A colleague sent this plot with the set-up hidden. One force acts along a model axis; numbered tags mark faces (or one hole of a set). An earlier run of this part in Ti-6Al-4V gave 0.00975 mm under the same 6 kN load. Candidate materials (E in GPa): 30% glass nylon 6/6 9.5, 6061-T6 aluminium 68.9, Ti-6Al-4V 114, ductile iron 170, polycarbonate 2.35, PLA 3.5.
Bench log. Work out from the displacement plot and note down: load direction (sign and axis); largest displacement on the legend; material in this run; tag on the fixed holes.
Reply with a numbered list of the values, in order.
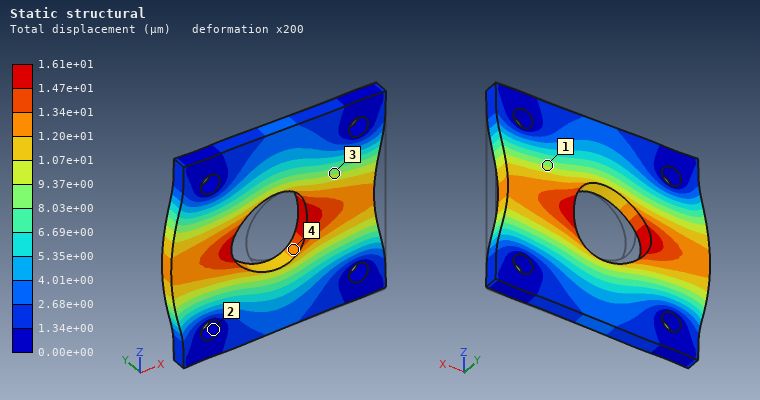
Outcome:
1. -X
2. 1.61e+01 µm
3. 6061-T6 aluminium
4. 2
